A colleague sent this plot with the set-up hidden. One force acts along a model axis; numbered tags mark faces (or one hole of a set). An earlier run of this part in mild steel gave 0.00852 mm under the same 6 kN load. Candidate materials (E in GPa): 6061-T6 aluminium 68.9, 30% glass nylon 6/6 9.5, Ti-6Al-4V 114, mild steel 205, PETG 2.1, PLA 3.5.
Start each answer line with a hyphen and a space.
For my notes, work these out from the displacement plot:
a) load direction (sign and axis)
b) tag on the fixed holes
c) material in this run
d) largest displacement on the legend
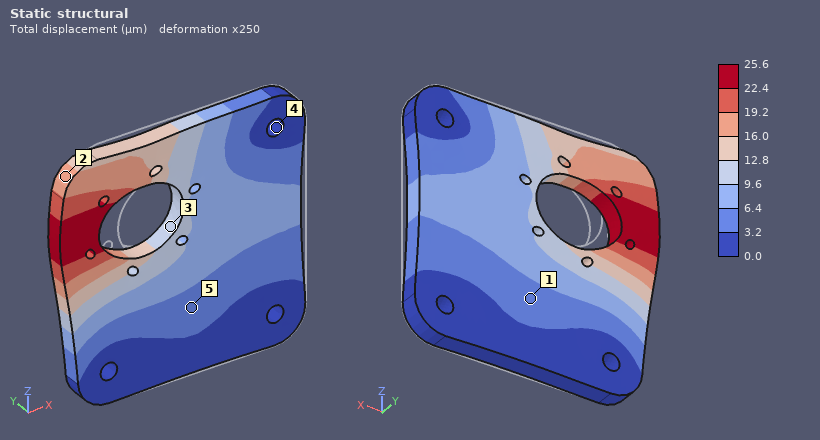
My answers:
- -X
- 4
- 6061-T6 aluminium
- 25.6 µm
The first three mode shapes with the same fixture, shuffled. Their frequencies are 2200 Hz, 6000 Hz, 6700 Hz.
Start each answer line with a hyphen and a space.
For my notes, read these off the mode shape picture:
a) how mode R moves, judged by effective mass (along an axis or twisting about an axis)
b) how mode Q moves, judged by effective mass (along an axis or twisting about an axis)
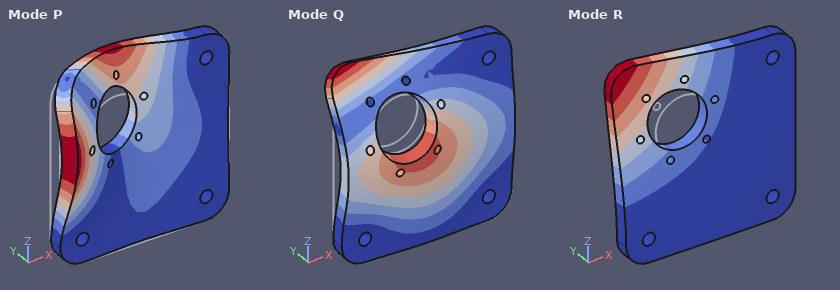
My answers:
- along Y
- along Y
